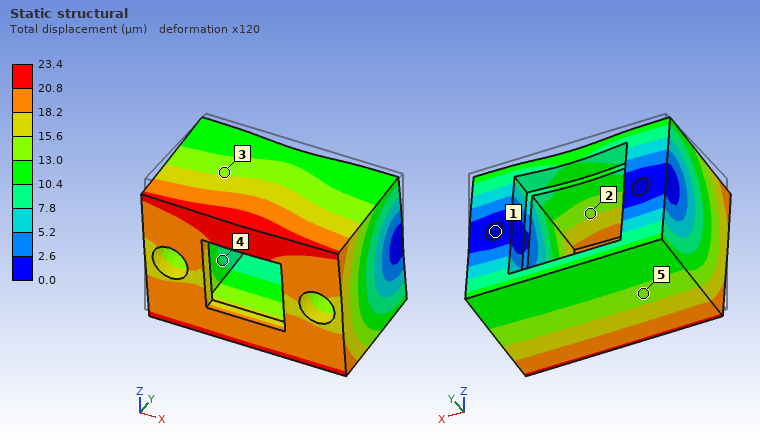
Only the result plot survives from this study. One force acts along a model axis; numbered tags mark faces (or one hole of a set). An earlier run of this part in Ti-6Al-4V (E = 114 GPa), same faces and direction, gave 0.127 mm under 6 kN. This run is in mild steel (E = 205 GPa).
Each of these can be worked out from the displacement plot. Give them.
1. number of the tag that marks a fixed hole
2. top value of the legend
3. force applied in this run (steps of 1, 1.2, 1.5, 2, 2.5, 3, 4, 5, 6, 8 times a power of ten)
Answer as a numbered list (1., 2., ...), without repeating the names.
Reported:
1. 1
2. 23.4 µm
3. 2 kN
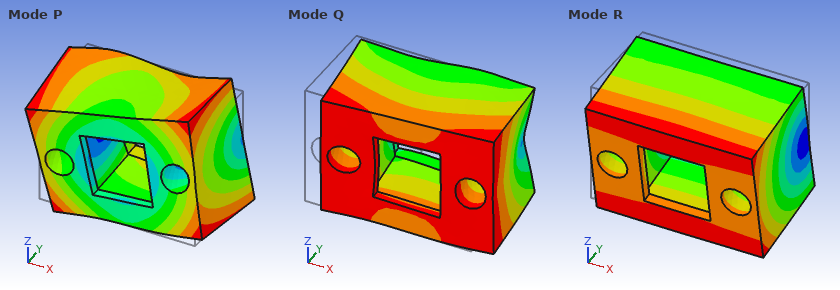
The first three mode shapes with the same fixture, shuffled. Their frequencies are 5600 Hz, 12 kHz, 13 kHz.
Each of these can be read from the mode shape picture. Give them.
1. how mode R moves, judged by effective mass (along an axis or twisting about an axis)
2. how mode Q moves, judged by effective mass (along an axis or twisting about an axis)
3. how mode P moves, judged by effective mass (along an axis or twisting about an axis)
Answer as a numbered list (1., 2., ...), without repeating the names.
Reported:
1. along Z
2. along X
3. twisting about Y
